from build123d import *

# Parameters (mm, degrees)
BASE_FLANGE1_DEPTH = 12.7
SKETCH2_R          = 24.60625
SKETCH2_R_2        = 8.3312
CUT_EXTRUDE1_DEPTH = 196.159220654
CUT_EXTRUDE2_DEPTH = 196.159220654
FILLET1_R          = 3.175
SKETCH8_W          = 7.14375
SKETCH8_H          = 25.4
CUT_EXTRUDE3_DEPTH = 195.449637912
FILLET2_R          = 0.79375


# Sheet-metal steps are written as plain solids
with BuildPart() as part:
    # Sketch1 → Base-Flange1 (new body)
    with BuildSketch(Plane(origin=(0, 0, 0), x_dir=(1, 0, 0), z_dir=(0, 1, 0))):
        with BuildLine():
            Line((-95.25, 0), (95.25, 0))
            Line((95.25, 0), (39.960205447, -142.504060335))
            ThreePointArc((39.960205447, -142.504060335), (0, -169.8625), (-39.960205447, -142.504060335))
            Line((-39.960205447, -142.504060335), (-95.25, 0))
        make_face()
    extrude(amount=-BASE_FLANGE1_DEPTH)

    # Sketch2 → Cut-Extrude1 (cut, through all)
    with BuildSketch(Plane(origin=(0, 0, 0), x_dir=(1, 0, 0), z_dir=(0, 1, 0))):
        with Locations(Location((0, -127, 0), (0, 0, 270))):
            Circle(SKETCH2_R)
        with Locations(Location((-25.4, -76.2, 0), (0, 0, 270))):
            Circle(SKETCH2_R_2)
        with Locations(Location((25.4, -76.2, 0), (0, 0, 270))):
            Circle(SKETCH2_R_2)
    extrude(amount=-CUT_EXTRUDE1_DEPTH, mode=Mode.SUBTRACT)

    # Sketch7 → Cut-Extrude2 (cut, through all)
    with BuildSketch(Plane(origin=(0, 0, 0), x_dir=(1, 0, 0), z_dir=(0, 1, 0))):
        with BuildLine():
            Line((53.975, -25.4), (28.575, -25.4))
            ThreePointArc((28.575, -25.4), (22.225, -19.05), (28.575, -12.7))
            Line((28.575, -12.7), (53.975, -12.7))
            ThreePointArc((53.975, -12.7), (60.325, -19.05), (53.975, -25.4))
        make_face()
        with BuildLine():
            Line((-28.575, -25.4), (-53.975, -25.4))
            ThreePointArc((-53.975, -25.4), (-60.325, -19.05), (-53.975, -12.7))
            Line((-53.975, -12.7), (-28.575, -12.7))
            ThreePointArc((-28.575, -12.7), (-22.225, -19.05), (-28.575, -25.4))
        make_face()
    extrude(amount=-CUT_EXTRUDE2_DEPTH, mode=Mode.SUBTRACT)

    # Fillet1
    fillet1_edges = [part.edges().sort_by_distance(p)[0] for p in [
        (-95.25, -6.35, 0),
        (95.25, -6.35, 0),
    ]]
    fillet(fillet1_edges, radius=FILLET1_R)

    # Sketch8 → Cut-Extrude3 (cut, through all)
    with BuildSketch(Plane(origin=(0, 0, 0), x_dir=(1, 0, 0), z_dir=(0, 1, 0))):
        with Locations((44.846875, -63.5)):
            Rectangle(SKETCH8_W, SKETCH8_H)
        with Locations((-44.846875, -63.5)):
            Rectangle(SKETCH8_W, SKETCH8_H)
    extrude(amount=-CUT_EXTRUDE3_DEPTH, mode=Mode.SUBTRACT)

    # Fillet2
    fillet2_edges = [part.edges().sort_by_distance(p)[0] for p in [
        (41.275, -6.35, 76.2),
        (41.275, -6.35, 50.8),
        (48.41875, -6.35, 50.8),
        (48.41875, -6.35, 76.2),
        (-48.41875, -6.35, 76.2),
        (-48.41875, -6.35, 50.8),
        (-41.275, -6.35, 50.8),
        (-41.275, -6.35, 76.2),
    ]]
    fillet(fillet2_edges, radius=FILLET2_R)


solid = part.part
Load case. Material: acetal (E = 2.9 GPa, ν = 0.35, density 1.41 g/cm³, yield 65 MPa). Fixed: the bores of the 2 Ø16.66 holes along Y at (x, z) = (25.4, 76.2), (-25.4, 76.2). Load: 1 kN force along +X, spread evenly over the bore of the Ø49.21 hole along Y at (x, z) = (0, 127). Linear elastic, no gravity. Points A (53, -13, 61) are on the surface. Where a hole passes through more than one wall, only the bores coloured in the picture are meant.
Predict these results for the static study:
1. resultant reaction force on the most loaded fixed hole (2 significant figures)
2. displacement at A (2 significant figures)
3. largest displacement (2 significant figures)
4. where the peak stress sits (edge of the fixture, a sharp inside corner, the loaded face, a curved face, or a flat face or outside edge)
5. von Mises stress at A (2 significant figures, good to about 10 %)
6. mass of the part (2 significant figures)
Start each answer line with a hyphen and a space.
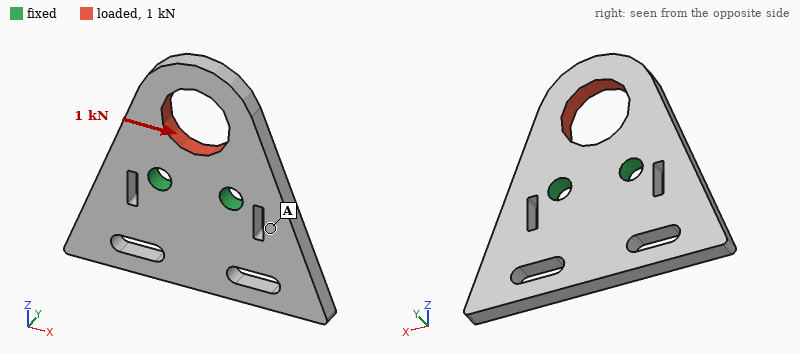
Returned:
- 860 N
- 0.030 mm
- 0.18 mm
- a curved face
- 0.63 MPa
- 310 g
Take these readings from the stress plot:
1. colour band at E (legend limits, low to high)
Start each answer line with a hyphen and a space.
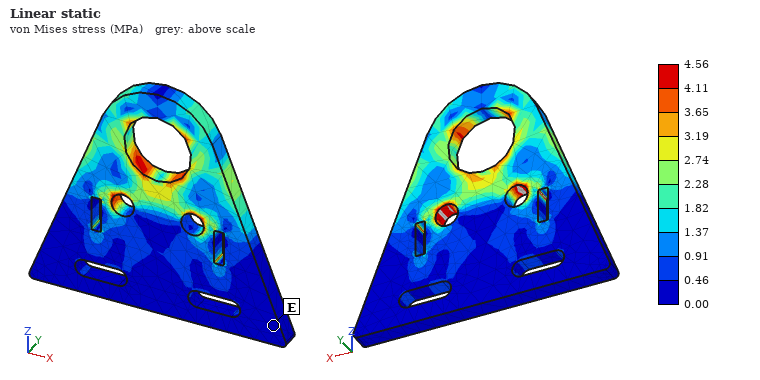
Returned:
- 0.00 to 0.46 MPa
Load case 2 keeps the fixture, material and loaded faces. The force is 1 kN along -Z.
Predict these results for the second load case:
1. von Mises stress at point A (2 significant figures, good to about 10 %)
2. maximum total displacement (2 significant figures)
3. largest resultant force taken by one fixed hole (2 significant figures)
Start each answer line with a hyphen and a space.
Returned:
- 0.26 MPa
- 50 µm
- 510 N
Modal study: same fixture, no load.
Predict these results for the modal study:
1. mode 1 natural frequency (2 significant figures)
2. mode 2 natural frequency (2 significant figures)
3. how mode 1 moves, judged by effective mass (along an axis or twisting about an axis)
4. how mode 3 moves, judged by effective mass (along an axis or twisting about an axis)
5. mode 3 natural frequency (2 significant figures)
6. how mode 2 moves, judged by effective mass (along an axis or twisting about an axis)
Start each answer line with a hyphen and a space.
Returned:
- 420 Hz
- 450 Hz
- along Y
- along Y
- 480 Hz
- twisting about Z
